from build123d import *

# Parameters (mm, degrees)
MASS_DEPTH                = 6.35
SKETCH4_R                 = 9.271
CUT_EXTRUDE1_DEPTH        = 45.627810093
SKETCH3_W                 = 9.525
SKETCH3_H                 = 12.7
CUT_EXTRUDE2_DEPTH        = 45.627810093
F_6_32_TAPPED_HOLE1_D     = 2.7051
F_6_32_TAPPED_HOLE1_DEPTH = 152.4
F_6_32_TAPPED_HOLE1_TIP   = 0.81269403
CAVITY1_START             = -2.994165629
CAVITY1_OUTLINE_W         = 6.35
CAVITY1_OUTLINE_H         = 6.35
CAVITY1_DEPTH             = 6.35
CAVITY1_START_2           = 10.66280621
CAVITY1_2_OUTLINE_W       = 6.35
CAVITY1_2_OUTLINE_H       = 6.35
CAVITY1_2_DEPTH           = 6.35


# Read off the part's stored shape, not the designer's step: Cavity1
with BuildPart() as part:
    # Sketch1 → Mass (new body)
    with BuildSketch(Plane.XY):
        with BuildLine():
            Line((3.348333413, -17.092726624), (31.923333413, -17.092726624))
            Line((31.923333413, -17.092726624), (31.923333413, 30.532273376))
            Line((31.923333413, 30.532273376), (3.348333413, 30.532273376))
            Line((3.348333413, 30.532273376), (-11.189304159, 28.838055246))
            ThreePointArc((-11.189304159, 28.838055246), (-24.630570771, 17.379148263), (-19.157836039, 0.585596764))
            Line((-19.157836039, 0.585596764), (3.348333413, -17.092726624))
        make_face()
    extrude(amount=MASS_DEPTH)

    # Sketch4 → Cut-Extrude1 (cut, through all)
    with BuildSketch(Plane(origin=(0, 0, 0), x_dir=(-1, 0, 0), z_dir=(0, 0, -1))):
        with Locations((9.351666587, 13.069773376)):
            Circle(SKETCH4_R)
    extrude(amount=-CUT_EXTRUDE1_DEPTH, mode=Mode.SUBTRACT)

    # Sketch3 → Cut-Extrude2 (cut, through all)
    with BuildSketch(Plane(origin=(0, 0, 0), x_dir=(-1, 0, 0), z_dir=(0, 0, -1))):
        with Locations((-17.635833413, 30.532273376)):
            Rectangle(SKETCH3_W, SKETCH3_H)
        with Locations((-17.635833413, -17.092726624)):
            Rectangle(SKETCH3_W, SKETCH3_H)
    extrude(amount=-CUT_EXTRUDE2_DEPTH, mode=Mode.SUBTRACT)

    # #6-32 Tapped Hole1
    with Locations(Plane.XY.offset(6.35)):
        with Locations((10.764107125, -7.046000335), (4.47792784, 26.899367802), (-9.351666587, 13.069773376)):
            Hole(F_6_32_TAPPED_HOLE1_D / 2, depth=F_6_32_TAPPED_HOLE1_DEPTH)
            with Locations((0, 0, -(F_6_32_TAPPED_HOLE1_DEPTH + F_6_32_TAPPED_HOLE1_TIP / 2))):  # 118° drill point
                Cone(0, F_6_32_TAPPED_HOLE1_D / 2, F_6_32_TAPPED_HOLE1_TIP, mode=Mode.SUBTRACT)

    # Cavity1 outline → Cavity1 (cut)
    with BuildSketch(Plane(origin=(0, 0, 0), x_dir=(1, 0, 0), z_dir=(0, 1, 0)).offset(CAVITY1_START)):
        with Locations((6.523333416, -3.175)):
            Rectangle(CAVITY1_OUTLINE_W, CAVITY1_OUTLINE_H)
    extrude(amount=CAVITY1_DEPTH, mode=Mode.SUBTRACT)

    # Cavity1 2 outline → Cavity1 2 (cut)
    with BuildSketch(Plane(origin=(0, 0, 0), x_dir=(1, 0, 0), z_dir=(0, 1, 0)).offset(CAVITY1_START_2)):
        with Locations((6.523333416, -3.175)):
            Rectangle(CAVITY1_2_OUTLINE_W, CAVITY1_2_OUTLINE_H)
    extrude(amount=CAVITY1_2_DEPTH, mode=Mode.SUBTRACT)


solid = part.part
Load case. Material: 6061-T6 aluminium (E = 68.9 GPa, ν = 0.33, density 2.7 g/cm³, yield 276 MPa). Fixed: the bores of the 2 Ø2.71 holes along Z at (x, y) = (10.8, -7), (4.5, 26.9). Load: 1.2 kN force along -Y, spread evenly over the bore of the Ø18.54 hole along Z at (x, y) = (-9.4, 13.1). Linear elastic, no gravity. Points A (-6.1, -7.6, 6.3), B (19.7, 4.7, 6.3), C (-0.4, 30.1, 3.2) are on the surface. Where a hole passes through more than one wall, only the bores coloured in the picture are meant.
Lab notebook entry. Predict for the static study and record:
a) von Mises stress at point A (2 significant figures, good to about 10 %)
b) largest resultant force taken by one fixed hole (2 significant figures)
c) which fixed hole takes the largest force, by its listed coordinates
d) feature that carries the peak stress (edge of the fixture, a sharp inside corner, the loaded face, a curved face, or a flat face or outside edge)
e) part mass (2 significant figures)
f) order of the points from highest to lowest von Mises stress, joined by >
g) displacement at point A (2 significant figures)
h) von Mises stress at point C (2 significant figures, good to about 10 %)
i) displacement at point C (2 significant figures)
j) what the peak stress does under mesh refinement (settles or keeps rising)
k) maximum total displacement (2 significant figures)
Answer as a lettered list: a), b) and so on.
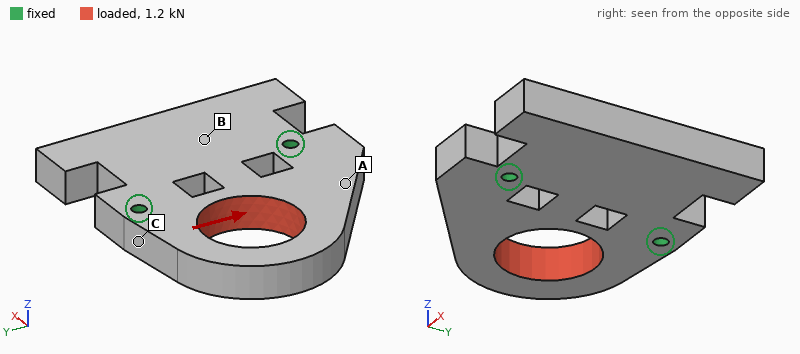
a) 10 MPa
b) 930 N
c) (4.5, 26.9)
d) edge of the fixture
e) 31 g
f) C > A > B
g) 7.8 µm
h) 21 MPa
i) 3.8 µm
j) keeps rising
k) 17 µm
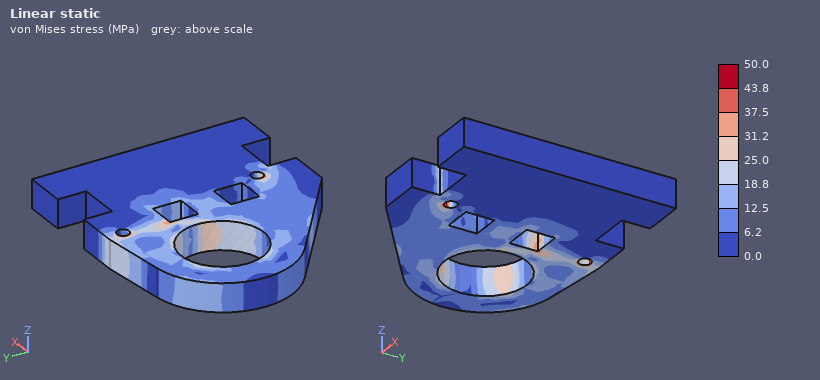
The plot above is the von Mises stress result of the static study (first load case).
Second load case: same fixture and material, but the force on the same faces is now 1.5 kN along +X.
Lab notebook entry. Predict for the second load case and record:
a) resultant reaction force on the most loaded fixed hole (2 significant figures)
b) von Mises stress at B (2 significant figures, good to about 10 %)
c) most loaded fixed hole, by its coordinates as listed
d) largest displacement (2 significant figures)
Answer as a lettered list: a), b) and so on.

a) 890 N
b) 3.1 MPa
c) (4.5, 26.9)
d) 6.2 µm
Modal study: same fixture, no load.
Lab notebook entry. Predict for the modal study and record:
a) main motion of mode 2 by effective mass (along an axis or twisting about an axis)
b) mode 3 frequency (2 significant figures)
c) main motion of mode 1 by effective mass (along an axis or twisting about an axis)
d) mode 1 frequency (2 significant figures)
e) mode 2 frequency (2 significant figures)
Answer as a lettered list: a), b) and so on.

a) along Z
b) 10 kHz
c) twisting about Y
d) 4800 Hz
e) 6200 Hz
